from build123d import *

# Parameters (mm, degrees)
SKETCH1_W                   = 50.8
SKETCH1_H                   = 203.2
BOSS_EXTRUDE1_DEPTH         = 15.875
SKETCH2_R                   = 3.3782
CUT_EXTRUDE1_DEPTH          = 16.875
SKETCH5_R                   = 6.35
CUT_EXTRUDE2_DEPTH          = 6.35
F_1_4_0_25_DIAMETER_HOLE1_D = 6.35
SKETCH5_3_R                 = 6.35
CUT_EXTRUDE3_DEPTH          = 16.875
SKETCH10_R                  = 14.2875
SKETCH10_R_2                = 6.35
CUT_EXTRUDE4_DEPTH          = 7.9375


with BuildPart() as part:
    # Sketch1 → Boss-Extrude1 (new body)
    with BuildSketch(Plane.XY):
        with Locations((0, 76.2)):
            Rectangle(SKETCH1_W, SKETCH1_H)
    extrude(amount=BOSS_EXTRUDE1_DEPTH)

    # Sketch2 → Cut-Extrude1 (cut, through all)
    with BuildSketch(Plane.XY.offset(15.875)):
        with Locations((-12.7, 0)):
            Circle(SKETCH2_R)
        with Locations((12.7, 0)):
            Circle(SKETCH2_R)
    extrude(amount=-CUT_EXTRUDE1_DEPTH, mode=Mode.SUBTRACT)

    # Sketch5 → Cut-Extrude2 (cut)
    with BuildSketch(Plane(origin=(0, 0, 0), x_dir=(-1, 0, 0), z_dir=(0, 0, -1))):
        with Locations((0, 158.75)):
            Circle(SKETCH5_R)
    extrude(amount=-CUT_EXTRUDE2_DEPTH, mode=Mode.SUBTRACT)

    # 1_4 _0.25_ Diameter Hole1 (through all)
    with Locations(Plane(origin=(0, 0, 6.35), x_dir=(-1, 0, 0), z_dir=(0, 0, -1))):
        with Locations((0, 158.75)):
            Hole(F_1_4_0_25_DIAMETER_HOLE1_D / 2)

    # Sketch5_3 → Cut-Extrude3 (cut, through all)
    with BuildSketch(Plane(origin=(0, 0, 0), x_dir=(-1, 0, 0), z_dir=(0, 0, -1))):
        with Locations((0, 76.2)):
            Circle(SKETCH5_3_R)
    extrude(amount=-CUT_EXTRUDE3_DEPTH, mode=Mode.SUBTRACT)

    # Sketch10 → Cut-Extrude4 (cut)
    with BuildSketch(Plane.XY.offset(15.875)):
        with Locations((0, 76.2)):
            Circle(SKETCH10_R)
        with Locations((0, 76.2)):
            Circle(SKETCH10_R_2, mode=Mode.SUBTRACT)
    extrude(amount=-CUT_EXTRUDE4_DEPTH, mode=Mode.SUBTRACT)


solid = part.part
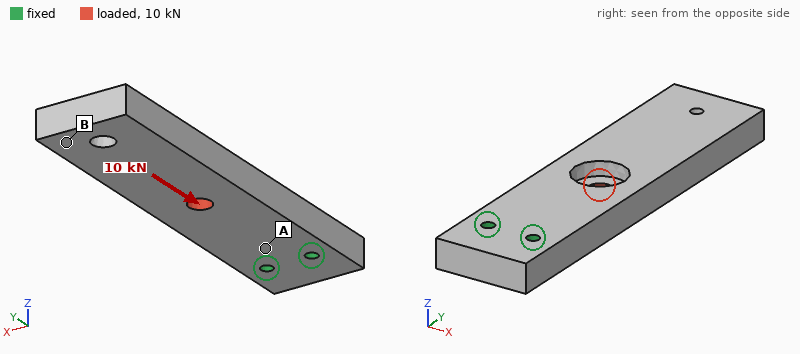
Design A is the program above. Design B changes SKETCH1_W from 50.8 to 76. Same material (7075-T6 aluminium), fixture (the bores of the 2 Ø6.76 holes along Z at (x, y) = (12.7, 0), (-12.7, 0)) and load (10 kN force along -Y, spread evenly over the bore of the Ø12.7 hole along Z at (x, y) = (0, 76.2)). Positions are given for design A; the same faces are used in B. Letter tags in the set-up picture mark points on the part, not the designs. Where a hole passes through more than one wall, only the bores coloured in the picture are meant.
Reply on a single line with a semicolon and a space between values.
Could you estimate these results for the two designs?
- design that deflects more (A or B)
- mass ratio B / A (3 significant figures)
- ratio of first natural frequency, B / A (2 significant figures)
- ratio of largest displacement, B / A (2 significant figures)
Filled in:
A; 1.52; 0.99; 0.69
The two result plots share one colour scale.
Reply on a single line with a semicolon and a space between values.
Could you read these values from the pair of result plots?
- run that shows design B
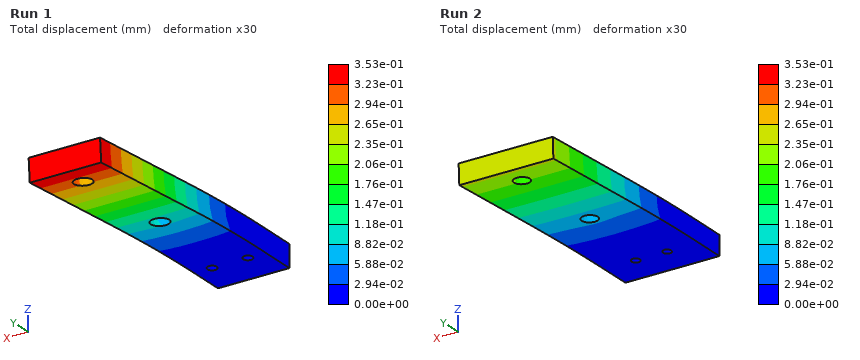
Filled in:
Run 2
